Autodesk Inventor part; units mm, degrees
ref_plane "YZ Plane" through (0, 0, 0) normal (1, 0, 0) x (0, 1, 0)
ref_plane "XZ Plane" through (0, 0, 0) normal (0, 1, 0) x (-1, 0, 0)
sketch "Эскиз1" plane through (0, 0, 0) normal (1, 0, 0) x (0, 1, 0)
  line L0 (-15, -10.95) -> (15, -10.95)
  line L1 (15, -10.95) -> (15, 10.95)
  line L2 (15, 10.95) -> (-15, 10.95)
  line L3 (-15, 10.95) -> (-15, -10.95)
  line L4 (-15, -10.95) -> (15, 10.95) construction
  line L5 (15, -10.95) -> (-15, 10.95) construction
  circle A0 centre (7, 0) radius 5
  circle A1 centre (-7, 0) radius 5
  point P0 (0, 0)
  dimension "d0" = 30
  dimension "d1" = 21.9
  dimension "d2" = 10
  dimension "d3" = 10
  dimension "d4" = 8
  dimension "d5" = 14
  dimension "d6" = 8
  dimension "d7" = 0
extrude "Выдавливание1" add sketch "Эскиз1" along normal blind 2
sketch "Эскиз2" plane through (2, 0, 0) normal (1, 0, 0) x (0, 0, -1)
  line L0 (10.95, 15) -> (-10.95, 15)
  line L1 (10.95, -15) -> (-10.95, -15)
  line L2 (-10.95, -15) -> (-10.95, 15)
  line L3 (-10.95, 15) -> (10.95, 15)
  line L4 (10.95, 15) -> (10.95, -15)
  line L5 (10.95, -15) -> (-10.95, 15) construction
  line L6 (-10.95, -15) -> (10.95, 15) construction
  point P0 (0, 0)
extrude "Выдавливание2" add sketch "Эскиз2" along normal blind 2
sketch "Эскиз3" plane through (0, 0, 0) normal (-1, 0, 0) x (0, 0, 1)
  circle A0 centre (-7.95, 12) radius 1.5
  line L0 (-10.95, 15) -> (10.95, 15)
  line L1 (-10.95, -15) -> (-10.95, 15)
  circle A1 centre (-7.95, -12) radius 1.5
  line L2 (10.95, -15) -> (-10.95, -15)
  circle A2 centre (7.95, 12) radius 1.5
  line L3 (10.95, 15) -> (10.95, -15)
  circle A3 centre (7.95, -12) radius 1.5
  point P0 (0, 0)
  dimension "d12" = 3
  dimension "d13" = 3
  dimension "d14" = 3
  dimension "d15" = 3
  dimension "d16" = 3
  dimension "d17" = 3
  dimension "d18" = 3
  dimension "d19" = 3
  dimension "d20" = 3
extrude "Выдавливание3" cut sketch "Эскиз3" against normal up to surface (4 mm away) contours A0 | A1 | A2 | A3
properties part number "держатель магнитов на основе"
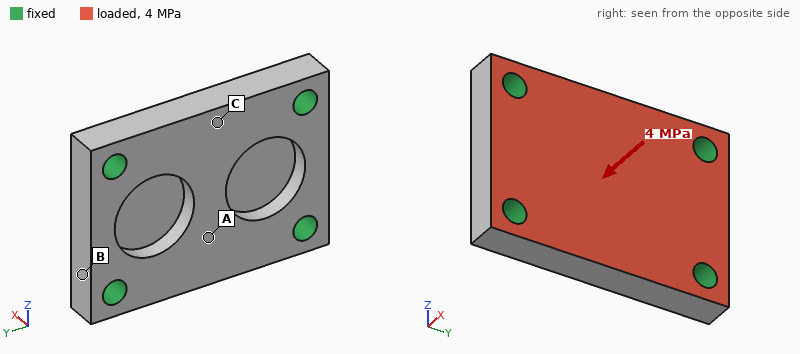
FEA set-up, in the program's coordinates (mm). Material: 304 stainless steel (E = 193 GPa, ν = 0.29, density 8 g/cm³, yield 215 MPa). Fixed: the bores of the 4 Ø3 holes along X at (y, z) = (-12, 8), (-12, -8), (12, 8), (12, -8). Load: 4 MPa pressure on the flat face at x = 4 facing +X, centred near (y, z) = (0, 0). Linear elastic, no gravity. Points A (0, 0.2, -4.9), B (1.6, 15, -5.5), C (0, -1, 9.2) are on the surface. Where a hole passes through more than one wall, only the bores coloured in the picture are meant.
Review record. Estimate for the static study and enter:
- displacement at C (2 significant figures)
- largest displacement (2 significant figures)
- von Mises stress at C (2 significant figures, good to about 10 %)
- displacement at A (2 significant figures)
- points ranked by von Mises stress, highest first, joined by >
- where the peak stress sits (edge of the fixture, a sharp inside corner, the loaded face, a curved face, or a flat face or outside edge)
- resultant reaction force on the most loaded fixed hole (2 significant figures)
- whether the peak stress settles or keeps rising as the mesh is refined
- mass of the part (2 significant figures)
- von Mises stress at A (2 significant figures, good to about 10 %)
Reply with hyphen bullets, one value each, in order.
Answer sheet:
- 4.6 µm
- 6.7 µm
- 42 MPa
- 5.7 µm
- C > A > B
- edge of the fixture
- 640 N
- keeps rising
- 18 g
- 33 MPa
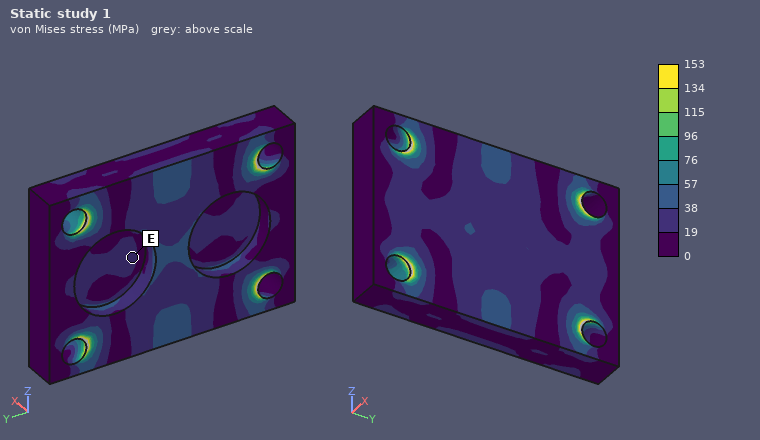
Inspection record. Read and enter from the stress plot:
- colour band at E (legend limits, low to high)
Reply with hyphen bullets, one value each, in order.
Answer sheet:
- 19 to 38 MPa
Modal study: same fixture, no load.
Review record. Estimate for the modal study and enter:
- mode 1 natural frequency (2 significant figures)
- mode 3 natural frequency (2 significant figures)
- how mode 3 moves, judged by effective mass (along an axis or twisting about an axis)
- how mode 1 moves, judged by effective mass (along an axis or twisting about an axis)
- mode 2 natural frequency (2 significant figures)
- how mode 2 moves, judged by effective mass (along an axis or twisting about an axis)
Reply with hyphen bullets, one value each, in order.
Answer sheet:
- 28 kHz
- 52 kHz
- along Z
- along X
- 37 kHz
- twisting about Y
